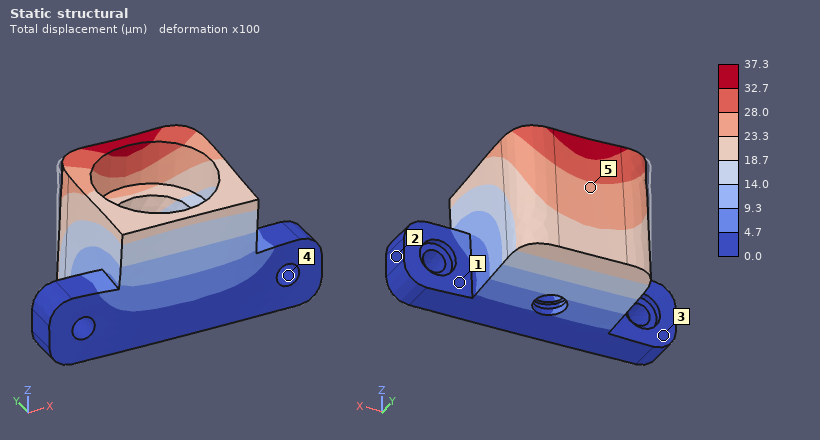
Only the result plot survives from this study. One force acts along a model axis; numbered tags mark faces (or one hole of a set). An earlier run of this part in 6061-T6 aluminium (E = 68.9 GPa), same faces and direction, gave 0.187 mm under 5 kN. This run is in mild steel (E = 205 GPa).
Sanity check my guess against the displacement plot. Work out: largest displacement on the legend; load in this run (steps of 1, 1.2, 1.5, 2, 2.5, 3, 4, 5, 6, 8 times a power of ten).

37.3 µm
3 kN
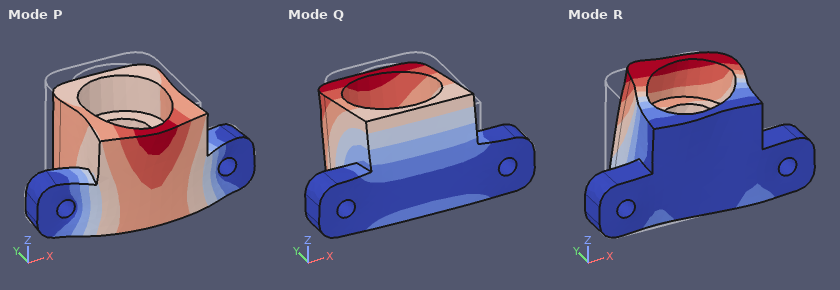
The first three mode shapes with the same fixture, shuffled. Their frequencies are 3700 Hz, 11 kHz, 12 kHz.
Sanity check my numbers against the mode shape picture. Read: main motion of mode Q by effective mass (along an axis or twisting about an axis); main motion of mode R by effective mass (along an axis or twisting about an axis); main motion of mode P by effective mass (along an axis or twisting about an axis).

along Z
along X
along Y
